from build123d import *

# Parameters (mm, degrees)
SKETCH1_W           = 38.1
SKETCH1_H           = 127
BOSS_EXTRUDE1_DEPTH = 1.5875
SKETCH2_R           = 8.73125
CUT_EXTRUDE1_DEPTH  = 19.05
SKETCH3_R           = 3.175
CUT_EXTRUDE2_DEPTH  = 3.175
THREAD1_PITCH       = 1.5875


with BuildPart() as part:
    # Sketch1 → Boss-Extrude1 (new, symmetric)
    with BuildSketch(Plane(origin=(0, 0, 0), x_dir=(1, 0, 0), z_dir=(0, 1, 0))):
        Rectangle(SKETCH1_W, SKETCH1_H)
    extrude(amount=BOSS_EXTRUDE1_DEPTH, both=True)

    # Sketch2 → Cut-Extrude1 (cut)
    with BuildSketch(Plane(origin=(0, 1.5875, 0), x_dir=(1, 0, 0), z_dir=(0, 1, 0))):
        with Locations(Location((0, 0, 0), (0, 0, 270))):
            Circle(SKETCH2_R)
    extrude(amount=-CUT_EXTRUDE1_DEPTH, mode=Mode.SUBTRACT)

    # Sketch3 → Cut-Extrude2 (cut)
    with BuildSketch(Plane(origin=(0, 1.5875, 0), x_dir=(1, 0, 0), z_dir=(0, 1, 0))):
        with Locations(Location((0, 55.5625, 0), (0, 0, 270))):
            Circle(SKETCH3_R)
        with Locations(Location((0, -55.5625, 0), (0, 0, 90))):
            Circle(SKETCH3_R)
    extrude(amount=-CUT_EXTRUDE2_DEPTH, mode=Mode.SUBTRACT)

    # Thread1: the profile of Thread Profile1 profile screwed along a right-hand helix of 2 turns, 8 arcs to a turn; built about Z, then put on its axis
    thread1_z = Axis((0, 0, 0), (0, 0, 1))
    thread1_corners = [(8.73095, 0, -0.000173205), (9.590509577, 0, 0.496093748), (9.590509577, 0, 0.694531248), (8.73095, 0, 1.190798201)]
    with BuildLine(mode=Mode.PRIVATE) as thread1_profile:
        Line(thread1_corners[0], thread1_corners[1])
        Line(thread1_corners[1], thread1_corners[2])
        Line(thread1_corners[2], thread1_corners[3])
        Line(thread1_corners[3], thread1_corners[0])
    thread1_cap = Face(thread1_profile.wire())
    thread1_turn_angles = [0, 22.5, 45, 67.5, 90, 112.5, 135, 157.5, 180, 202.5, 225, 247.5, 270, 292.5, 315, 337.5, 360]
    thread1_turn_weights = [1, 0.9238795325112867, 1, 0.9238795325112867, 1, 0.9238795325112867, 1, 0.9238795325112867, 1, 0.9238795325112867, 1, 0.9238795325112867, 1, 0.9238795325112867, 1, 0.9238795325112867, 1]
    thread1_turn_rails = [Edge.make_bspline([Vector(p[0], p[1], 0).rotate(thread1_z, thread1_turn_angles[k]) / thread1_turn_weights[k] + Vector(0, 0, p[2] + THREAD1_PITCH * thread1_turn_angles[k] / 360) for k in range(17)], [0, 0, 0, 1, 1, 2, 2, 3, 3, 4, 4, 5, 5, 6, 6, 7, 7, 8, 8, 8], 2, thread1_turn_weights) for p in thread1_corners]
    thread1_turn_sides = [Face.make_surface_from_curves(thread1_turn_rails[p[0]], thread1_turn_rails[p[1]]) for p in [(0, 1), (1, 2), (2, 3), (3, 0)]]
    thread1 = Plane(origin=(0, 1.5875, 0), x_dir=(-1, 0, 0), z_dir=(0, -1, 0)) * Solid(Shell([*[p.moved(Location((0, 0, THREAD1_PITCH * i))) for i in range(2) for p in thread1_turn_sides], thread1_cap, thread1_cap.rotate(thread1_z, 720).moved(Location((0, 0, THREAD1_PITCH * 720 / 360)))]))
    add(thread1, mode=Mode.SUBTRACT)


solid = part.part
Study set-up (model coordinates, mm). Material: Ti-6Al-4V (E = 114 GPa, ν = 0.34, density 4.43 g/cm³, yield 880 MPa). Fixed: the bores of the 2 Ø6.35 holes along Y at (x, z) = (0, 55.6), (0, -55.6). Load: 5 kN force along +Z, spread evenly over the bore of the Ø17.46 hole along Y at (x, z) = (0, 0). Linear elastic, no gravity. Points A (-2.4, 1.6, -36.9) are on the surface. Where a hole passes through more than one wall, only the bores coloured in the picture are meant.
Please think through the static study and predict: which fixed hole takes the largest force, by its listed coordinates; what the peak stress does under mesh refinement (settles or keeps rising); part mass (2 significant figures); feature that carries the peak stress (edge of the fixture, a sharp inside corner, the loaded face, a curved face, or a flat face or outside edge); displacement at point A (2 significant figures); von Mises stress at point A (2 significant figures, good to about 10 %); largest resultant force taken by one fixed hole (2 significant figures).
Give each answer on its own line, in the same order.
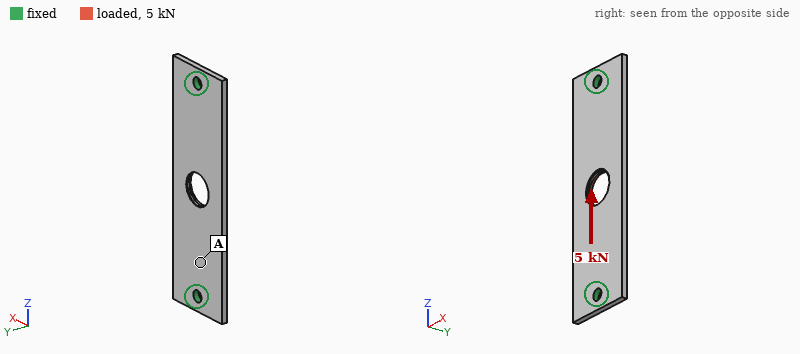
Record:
(0, 55.6)
keeps rising
64 g
a sharp inside corner
8.4 µm
24 MPa
2.8 kN
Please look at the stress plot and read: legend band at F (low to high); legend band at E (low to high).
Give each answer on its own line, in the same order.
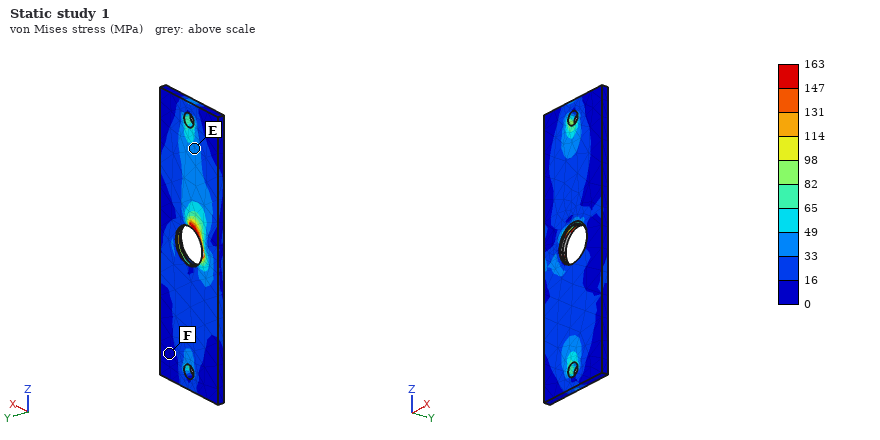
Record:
0 to 16 MPa
33 to 49 MPa
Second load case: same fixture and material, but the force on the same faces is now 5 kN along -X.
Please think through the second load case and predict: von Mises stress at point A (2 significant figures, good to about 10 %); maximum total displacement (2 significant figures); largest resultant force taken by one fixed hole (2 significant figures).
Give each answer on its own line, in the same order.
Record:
58 MPa
0.11 mm
2.6 kN
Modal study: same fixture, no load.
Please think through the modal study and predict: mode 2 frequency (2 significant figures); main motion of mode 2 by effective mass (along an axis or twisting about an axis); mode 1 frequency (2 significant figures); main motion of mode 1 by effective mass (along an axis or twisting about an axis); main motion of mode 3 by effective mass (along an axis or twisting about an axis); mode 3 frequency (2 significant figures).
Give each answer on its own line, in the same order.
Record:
2300 Hz
twisting about Z
1400 Hz
along Y
twisting about X
3500 Hz
